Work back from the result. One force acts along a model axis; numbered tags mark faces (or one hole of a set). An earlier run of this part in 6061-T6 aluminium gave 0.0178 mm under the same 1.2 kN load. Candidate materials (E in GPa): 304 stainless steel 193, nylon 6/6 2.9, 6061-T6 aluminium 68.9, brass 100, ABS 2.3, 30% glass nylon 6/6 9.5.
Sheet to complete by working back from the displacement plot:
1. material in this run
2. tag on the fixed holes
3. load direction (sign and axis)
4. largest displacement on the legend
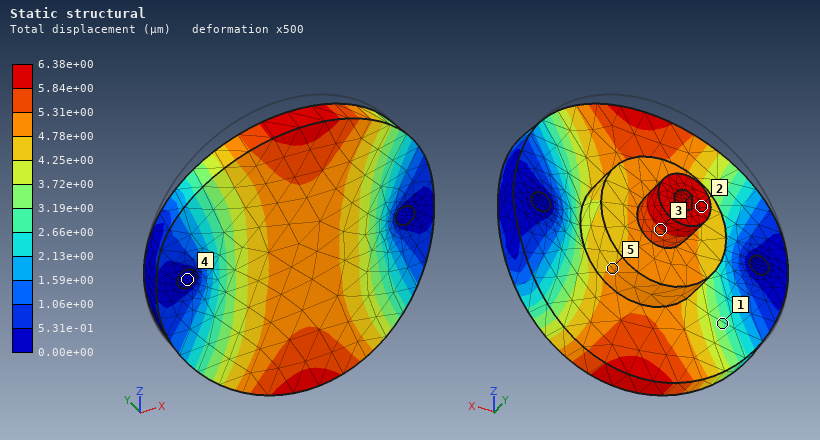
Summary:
304 stainless steel
4
-Y
6.38e+00 µm
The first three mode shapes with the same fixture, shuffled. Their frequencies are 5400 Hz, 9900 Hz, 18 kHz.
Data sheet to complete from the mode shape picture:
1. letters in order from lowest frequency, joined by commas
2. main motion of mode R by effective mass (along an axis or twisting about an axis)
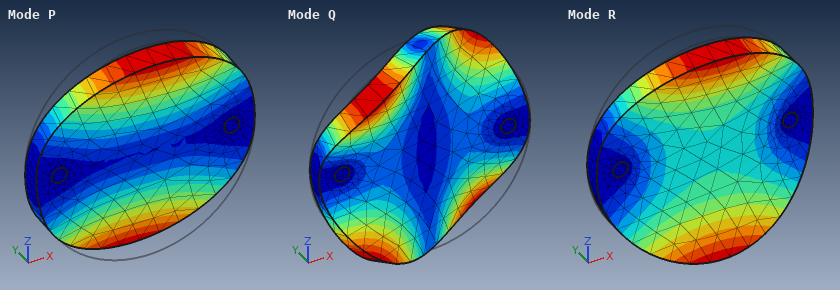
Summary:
P, R, Q
along Y
